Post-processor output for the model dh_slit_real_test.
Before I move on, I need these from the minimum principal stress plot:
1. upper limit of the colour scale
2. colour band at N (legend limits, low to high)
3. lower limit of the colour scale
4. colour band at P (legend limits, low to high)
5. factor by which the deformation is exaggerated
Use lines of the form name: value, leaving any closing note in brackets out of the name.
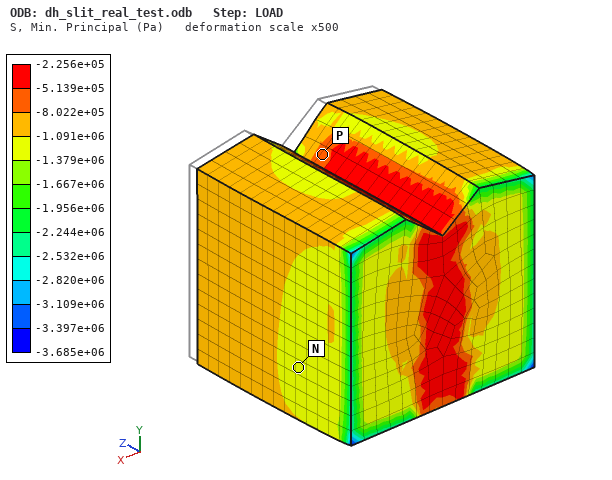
upper limit of the colour scale: -2.256e+05 Pa
colour band at N: -1.379e+06 to -1.091e+06 Pa
lower limit of the colour scale: -3.685e+06 Pa
colour band at P: -8.022e+05 to -5.139e+05 Pa
factor by which the deformation is exaggerated: 500
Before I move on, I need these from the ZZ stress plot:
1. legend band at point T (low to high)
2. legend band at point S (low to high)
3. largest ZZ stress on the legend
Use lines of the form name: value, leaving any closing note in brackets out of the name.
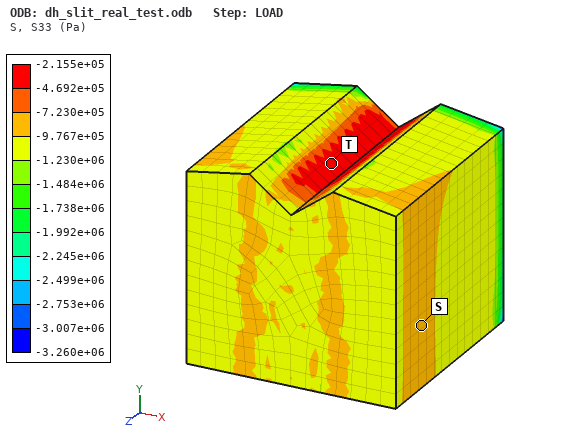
legend band at point T: -4.692e+05 to -2.155e+05 Pa
legend band at point S: -9.767e+05 to -7.230e+05 Pa
largest ZZ stress on the legend: -2.155e+05 Pa
